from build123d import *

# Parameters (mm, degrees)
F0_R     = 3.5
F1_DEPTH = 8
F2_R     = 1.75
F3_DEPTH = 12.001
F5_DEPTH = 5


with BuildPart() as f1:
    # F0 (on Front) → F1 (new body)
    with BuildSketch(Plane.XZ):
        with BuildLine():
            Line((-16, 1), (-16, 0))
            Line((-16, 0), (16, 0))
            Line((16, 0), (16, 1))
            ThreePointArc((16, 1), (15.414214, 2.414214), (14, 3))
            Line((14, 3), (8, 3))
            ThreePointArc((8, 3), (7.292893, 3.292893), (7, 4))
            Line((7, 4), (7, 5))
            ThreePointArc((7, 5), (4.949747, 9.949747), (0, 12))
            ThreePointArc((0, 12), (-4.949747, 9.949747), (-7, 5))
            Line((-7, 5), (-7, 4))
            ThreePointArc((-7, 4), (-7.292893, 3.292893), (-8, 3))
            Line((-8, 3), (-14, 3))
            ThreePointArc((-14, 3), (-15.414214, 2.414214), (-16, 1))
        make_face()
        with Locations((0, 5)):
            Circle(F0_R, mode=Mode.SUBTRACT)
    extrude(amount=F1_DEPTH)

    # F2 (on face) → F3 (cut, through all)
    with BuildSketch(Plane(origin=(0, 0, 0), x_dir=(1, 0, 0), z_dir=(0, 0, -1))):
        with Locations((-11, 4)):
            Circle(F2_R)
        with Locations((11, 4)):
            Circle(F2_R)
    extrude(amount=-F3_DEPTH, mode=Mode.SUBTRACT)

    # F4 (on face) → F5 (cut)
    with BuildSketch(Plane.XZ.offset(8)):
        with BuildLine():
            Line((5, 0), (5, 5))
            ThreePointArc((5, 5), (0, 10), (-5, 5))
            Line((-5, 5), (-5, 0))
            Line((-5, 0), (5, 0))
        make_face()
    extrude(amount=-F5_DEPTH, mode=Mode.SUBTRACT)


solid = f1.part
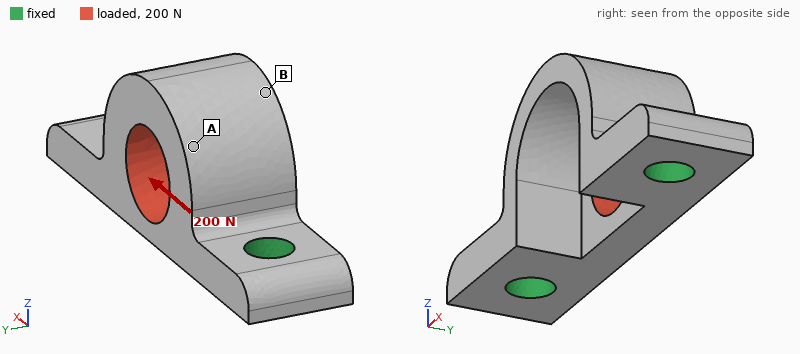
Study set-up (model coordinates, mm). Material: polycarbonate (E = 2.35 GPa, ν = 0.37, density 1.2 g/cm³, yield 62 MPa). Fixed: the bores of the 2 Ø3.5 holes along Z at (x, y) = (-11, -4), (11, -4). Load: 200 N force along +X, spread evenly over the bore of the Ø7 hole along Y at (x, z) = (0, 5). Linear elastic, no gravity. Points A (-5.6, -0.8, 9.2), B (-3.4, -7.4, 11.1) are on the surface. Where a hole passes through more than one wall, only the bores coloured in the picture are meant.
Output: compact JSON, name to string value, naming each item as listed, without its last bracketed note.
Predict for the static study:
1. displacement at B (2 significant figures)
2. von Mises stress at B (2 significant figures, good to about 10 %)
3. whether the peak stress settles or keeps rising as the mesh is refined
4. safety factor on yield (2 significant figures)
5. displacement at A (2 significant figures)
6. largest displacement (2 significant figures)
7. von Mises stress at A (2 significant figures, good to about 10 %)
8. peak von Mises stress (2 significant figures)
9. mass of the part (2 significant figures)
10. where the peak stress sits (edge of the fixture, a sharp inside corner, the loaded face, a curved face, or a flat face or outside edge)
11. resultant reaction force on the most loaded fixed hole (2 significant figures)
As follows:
{"displacement at B": "60 µm", "von Mises stress at B": "3.6 MPa", "whether the peak stress settles or keeps rising as the mesh is refined": "settles", "safety factor on yield": "2.4", "displacement at A": "77 µm", "largest displacement": "82 µm", "von Mises stress at A": "7.3 MPa", "peak von Mises stress": "26 MPa", "mass of the part": "1.2 g", "where the peak stress sits": "a curved face", "resultant reaction force on the most loaded fixed hole": "110 N"}
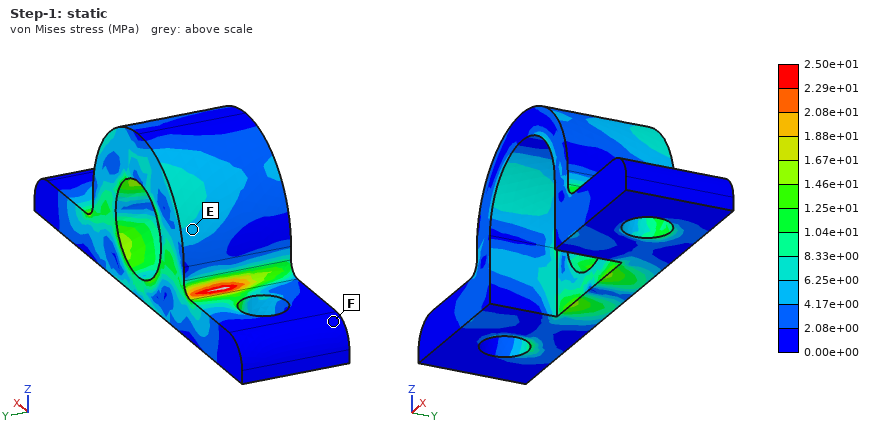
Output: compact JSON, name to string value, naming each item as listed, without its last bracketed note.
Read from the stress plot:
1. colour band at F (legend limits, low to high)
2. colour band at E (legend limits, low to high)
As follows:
{"colour band at F": "0.00e+00 to 2.08e+00 MPa", "colour band at E": "4.17e+00 to 6.25e+00 MPa"}
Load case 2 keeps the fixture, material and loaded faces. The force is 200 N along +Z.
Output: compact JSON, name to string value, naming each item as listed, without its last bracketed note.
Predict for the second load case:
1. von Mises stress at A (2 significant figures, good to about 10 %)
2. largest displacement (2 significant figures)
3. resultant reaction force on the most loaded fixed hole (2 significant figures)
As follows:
{"von Mises stress at A": "4.7 MPa", "largest displacement": "0.21 mm", "resultant reaction force on the most loaded fixed hole": "100 N"}
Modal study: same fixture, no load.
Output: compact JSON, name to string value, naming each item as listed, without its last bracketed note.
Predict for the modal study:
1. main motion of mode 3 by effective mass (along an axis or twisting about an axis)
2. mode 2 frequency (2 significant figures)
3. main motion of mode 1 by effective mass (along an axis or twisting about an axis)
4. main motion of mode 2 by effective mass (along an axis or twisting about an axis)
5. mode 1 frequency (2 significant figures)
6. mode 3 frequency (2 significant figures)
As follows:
{"main motion of mode 3 by effective mass": "along Z", "mode 2 frequency": "8600 Hz", "main motion of mode 1 by effective mass": "along Y", "main motion of mode 2 by effective mass": "along X", "mode 1 frequency": "4900 Hz", "mode 3 frequency": "11 kHz"}
